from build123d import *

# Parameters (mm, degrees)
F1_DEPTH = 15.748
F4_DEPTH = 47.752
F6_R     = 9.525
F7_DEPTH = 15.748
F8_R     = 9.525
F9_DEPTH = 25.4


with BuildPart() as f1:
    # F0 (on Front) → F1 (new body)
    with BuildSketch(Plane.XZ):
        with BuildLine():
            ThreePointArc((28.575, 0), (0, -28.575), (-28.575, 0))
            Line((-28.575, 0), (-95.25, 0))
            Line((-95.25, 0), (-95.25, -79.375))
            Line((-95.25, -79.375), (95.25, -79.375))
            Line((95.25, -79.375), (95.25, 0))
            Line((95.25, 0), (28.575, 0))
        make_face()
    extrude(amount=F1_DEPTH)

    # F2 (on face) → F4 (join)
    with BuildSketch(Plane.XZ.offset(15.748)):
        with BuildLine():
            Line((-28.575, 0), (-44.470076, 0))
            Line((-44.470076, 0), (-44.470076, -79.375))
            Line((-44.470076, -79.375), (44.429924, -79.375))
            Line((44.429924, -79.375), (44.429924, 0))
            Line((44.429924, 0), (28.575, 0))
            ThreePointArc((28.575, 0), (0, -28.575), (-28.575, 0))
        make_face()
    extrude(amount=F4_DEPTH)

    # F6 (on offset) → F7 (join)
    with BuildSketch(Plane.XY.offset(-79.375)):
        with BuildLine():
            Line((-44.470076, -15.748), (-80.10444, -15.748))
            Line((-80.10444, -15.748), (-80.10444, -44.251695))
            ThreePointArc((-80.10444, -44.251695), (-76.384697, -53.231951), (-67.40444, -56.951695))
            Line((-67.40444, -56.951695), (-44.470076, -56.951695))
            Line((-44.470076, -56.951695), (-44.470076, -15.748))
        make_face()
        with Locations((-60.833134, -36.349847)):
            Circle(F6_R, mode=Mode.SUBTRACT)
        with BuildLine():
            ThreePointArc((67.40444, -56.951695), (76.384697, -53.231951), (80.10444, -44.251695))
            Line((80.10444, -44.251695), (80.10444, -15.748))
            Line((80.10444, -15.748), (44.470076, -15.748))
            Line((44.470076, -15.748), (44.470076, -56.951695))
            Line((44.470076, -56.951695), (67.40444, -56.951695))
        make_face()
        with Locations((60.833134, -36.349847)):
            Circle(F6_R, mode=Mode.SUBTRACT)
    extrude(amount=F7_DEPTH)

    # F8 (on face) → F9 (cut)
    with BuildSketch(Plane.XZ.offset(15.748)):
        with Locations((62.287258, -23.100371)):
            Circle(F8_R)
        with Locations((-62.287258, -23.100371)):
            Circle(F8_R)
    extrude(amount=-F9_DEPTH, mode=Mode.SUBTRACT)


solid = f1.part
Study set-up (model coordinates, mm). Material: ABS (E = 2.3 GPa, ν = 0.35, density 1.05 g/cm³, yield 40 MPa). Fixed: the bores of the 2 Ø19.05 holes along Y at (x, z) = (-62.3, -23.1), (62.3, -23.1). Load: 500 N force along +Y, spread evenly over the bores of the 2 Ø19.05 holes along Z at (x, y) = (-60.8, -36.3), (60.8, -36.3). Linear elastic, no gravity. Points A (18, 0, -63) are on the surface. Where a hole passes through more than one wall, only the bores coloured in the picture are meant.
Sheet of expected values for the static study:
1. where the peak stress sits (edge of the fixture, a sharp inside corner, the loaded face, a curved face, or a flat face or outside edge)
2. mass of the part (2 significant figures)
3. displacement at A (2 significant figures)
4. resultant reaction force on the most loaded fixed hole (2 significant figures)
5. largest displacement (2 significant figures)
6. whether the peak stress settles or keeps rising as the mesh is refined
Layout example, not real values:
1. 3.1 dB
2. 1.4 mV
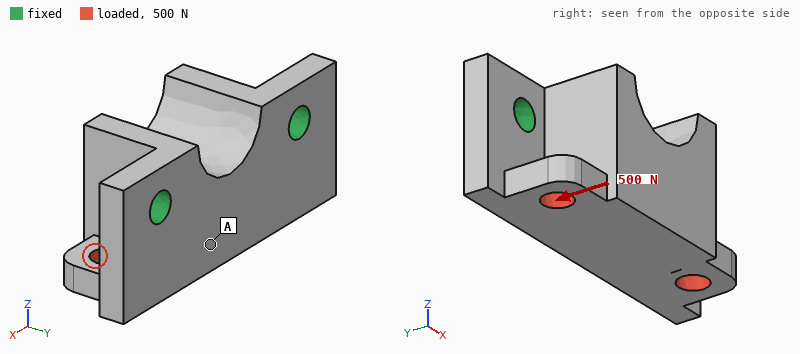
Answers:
1. a sharp inside corner
2. 550 g
3. 0.086 mm
4. 250 N
5. 0.21 mm
6. keeps rising
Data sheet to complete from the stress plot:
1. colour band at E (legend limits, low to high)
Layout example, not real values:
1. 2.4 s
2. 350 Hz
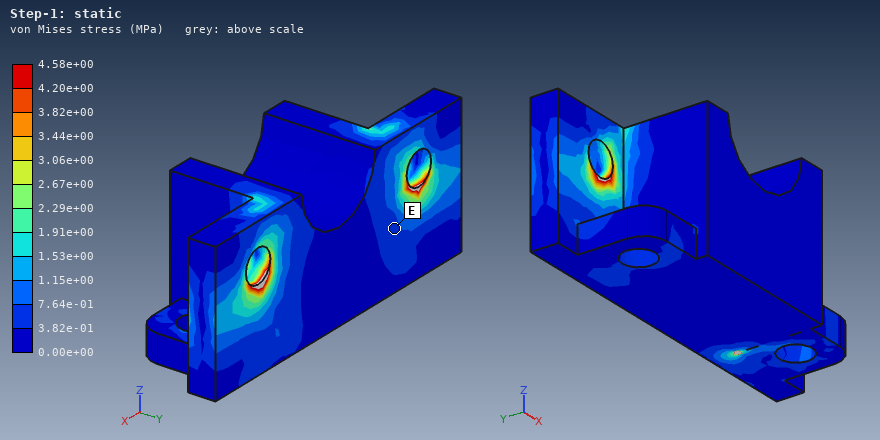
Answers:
1. 3.82e-01 to 7.64e-01 MPa
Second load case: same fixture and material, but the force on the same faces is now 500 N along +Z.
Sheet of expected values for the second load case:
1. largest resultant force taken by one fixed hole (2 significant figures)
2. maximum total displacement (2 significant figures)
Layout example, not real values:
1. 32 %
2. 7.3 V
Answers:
1. 260 N
2. 0.37 mm
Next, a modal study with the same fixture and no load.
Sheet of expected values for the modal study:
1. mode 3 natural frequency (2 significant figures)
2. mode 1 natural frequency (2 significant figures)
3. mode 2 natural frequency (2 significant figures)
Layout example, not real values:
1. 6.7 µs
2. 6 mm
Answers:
1. 1500 Hz
2. 530 Hz
3. 1100 Hz
